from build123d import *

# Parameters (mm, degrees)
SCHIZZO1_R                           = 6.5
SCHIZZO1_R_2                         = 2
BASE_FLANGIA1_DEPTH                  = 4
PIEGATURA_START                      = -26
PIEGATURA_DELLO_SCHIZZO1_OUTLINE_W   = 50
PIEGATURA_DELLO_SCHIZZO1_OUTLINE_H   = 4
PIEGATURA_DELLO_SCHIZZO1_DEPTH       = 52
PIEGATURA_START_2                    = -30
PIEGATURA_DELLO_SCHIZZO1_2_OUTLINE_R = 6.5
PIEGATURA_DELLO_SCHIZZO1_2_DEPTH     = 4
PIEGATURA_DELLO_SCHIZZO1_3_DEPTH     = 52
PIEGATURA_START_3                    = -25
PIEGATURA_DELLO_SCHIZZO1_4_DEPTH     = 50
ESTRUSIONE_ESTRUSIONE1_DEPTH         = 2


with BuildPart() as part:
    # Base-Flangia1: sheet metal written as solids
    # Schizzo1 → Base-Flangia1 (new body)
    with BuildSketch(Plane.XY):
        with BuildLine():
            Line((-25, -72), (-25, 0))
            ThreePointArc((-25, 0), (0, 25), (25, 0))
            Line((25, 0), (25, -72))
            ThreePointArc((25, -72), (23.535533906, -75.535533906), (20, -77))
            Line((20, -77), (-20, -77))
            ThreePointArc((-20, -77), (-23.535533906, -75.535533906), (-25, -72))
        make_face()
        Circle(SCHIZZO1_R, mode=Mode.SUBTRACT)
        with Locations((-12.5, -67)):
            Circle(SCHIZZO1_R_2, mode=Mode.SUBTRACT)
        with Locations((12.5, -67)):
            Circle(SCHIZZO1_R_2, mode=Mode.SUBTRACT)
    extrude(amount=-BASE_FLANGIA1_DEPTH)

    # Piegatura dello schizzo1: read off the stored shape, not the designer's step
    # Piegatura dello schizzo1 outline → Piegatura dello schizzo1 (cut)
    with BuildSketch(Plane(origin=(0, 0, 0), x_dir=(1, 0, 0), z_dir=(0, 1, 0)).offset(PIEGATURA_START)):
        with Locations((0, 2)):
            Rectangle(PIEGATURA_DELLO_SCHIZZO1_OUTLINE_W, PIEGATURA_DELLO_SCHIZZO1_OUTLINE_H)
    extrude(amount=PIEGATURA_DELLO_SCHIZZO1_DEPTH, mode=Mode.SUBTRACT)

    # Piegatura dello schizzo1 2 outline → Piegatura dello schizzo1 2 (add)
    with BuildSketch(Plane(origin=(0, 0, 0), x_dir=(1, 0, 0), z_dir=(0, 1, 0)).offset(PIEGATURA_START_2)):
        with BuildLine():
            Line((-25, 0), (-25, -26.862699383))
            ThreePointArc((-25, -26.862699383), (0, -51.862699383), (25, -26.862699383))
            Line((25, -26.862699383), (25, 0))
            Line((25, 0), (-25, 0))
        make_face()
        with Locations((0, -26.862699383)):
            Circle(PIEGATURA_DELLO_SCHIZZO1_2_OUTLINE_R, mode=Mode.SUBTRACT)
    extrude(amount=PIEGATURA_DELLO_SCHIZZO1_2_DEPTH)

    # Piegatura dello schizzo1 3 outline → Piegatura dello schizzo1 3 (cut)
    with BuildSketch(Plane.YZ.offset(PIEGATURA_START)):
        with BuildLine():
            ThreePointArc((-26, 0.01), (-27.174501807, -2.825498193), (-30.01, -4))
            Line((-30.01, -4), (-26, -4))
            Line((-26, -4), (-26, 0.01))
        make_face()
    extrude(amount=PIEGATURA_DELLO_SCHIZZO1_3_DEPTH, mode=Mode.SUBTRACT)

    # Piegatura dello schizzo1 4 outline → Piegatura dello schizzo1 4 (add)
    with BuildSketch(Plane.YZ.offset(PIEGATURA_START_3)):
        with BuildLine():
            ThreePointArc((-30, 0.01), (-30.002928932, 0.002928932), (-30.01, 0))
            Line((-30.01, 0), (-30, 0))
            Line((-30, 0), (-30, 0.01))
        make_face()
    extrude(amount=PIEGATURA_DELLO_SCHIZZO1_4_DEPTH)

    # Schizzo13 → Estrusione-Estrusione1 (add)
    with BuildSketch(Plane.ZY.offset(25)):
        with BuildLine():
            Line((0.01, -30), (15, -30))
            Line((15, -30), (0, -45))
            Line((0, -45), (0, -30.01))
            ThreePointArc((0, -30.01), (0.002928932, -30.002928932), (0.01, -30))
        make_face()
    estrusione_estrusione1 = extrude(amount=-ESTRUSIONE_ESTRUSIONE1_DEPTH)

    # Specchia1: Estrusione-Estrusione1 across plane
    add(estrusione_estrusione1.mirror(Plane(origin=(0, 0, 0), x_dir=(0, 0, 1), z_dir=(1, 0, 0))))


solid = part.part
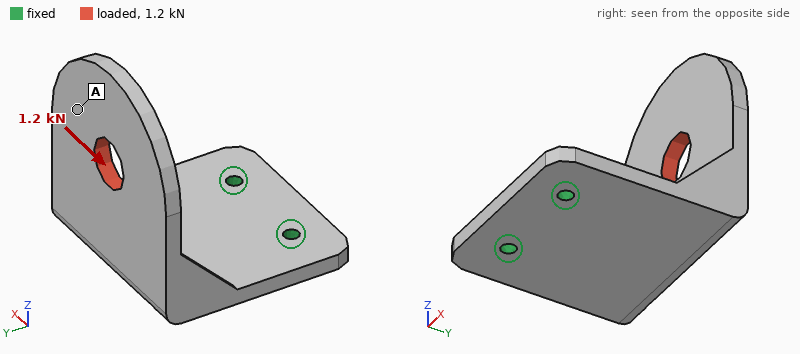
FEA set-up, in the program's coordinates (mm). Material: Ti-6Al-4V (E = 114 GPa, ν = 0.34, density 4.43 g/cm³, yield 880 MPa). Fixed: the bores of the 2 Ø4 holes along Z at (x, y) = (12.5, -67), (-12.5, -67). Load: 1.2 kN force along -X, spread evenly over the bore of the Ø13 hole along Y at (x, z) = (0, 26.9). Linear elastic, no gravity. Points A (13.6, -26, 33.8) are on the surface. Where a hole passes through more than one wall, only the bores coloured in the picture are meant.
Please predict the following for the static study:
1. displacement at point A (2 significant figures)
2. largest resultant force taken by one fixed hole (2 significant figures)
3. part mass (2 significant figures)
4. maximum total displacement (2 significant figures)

0.60 mm
2.1 kN
85 g
0.86 mm
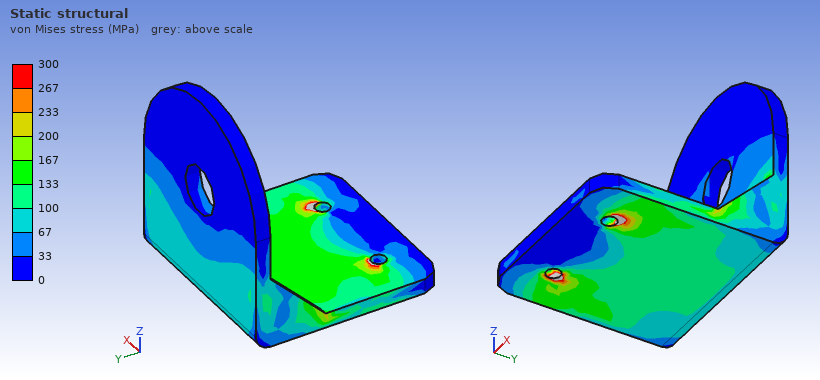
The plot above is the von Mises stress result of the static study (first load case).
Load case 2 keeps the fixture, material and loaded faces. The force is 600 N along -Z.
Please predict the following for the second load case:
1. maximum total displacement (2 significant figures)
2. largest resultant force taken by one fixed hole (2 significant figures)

0.87 mm
300 N
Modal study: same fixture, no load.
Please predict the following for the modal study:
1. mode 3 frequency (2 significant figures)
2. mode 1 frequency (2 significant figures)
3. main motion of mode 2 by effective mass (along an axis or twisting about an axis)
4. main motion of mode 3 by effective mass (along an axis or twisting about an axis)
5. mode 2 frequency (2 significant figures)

1900 Hz
610 Hz
along X
along Z
1100 Hz
